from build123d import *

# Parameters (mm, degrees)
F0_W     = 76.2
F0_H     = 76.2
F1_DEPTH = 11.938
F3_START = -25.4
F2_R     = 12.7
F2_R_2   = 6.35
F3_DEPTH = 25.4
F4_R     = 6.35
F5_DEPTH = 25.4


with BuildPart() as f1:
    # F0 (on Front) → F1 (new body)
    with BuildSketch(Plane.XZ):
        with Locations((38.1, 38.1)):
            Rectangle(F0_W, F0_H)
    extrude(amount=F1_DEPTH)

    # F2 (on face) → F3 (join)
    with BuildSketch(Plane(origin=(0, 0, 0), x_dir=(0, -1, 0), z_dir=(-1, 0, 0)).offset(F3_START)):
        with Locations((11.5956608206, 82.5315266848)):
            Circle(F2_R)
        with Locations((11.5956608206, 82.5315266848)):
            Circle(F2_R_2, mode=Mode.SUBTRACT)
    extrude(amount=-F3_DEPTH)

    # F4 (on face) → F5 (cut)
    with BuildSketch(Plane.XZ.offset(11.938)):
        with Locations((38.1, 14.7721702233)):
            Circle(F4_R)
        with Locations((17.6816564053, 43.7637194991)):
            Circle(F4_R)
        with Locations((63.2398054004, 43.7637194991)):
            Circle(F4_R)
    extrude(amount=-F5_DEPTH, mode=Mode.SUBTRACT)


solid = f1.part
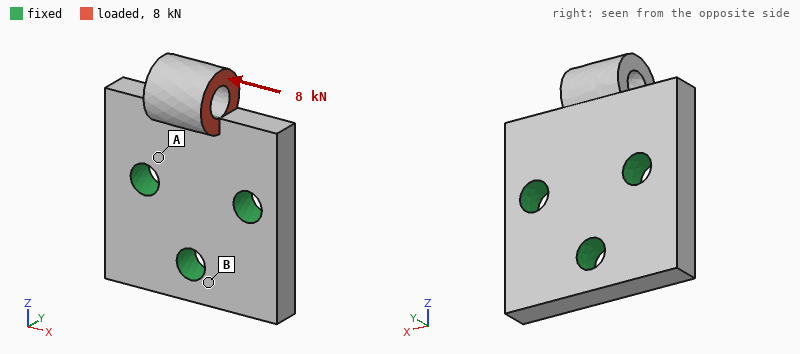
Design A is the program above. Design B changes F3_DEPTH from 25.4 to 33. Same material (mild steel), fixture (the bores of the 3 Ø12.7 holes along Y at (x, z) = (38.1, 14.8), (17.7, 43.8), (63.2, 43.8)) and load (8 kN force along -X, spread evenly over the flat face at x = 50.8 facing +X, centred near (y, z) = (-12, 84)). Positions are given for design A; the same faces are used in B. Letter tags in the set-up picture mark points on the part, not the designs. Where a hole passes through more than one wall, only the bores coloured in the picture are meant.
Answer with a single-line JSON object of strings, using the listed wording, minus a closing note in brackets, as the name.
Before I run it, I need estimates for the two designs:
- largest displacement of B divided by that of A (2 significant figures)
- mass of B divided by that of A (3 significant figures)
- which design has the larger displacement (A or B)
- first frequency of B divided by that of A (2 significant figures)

{"largest displacement of B divided by that of A": "0.74", "mass of B divided by that of A": "1.03", "which design has the larger displacement": "A", "first frequency of B divided by that of A": "0.93"}
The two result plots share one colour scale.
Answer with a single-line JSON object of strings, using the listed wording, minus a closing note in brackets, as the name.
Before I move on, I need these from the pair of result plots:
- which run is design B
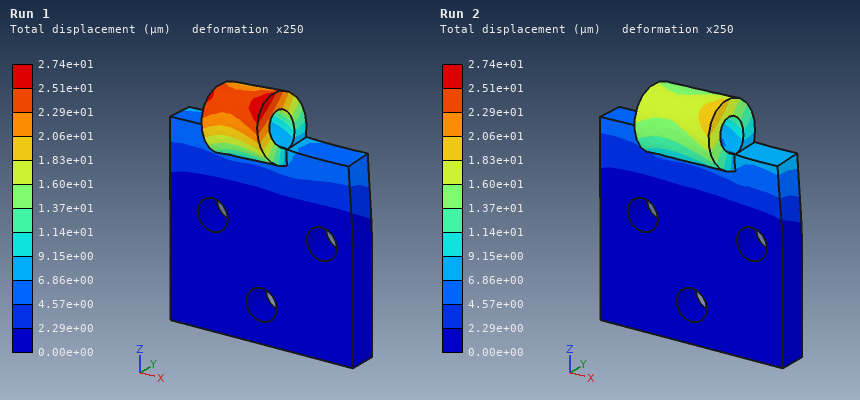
{"which run is design B": "Run 2"}
